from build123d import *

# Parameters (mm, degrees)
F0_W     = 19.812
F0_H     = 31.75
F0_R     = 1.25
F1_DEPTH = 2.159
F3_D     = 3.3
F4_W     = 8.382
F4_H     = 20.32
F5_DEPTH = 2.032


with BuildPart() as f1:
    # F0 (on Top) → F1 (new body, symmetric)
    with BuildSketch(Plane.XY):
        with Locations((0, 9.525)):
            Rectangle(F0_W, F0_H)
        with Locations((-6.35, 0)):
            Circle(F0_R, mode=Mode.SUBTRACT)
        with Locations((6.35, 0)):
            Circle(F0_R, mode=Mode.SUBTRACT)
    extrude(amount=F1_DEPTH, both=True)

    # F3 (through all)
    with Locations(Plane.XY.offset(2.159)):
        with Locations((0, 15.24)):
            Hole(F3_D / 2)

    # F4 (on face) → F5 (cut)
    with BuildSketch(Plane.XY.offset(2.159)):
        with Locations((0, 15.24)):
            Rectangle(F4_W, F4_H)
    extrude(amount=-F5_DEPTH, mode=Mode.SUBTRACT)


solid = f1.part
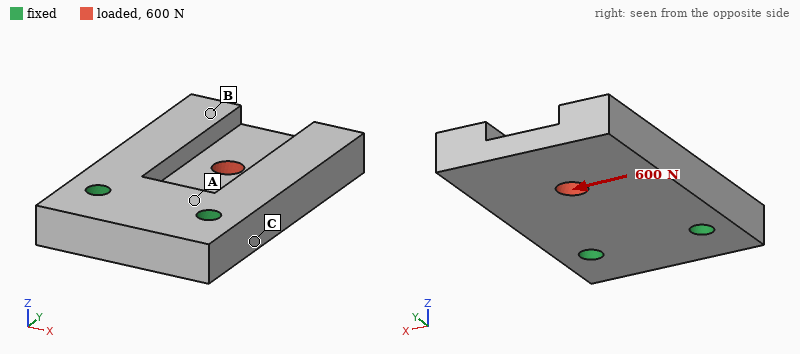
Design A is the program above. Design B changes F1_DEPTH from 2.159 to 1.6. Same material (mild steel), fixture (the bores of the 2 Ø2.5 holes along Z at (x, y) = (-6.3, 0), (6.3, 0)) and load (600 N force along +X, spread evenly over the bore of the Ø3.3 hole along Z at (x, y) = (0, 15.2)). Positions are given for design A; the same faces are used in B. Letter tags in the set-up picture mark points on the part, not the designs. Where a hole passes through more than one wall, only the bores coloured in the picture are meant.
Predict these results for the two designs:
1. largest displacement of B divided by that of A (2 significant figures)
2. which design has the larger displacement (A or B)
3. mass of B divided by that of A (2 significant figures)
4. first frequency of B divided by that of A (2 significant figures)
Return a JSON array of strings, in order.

["1.3", "B", "0.74", "0.76"]
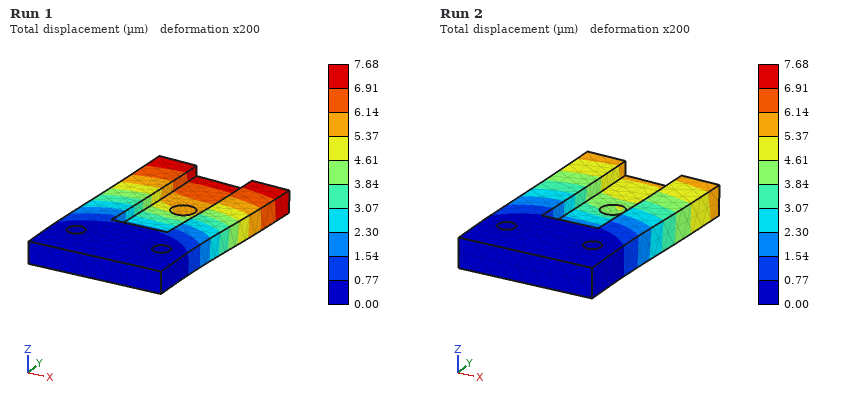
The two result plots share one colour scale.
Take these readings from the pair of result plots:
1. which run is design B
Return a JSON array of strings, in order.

["Run 1"]
